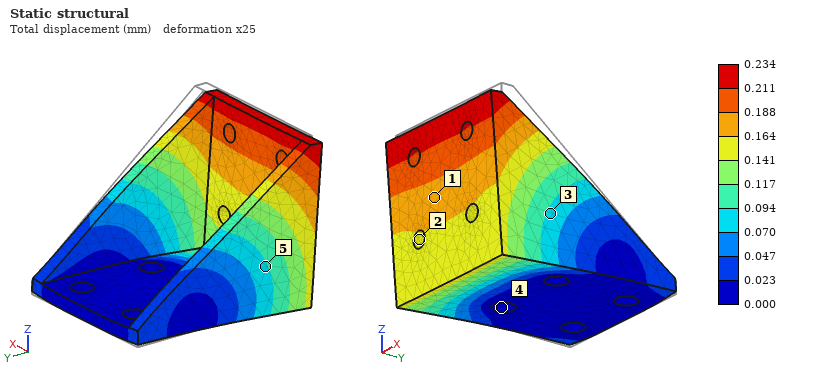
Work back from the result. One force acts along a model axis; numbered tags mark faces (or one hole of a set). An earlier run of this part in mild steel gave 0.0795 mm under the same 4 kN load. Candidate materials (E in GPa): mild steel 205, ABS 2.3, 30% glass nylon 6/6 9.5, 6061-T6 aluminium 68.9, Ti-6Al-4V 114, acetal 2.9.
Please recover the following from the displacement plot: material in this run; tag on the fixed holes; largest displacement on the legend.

6061-T6 aluminium
4
0.234 mm
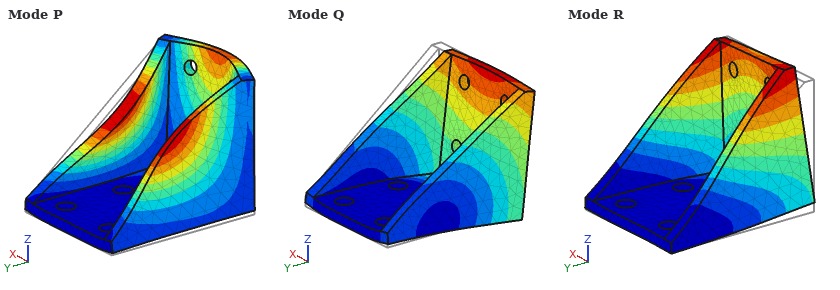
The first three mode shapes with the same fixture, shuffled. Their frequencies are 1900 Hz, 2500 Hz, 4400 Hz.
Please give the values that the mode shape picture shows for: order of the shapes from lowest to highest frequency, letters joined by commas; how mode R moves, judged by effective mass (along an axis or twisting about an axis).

R, Q, P
along X
